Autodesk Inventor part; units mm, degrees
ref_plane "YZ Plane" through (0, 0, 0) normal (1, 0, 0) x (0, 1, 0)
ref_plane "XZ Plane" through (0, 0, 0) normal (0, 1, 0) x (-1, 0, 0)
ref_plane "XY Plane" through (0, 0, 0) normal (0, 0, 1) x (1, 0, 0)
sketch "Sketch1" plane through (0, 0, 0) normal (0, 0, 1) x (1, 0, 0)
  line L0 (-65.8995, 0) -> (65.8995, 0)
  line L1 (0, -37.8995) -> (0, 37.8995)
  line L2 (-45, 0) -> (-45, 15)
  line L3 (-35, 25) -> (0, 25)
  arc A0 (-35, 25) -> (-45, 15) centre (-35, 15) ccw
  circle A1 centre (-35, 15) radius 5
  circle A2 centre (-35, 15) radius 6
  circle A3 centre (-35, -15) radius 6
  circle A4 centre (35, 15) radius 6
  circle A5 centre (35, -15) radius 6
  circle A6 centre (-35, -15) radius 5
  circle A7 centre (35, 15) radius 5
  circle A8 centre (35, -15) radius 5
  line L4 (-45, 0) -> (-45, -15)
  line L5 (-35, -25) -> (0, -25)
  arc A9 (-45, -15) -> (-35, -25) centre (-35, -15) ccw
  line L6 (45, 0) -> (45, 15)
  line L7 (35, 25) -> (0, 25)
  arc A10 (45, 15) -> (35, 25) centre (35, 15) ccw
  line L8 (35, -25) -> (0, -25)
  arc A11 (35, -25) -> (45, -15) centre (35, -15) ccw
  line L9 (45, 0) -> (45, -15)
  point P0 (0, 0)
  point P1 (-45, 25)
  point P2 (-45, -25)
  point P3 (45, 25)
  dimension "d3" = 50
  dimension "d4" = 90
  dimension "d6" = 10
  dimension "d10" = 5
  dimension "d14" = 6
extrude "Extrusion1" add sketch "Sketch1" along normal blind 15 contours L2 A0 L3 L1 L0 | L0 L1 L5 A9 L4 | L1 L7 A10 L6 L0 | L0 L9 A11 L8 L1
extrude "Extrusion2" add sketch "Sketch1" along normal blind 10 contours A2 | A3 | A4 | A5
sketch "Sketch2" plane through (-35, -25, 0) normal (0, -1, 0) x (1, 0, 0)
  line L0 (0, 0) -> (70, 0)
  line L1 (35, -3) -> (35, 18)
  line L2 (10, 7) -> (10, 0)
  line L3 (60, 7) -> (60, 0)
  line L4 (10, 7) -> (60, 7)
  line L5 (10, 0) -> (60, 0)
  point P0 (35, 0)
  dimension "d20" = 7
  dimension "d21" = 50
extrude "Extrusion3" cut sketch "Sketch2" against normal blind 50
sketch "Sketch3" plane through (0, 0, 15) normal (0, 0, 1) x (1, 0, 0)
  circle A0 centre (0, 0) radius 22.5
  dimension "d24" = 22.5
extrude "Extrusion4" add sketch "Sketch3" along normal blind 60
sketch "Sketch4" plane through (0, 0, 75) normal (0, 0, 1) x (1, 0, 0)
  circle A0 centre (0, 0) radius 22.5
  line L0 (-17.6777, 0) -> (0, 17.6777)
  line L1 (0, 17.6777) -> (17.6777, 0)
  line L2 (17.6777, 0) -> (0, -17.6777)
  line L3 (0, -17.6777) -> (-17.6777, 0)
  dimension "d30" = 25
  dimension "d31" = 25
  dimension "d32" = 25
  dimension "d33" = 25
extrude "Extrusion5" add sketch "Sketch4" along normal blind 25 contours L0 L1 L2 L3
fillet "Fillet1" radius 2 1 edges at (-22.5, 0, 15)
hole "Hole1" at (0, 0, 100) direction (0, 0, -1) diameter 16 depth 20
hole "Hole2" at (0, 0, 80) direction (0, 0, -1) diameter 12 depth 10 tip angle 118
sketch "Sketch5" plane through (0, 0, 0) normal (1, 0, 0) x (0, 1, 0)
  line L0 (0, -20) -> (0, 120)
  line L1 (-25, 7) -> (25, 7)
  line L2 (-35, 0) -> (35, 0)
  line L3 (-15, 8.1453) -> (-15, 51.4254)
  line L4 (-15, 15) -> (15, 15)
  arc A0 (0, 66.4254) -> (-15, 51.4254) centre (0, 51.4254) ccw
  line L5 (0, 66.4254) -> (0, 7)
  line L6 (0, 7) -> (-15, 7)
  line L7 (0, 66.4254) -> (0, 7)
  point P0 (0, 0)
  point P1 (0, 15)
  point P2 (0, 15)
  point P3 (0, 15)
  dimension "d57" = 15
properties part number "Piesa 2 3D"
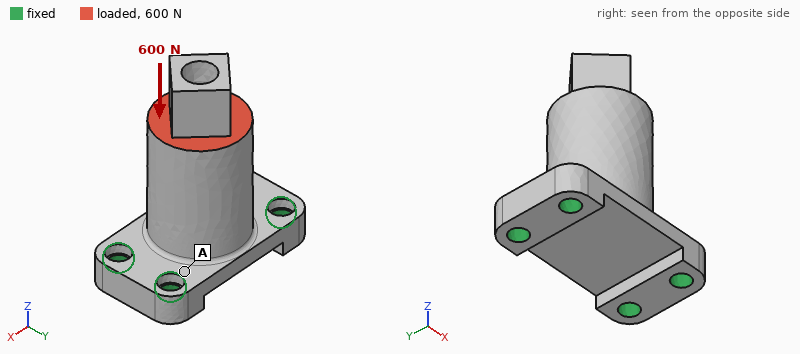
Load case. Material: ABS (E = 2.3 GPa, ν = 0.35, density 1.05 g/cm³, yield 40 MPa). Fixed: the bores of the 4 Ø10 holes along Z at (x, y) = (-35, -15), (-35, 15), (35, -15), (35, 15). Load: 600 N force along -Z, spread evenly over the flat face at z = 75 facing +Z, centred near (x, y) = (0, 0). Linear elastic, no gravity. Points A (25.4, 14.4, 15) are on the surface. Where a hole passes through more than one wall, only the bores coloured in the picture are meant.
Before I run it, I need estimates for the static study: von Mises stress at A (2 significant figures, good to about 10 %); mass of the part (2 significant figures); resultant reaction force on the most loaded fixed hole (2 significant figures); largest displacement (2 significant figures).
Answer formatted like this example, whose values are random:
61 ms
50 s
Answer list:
0.58 MPa
160 g
200 N
39 µm
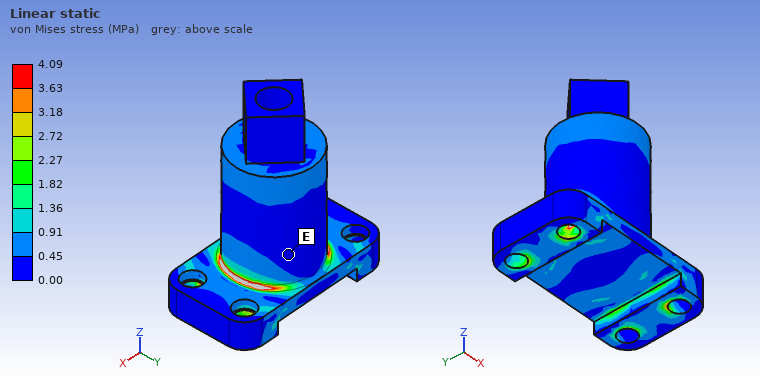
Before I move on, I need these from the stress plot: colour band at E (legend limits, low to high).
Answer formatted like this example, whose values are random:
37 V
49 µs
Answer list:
0.00 to 0.45 MPa
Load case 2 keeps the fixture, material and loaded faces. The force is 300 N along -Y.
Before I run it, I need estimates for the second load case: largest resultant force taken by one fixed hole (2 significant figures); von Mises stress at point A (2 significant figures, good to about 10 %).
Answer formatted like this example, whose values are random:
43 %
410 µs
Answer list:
400 N
4.0 MPa
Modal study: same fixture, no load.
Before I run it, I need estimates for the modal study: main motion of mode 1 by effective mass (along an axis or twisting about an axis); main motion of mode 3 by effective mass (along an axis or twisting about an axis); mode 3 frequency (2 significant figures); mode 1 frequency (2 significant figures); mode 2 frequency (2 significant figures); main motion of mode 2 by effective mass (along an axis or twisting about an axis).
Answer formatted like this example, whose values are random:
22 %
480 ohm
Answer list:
along Y
along Z
1900 Hz
590 Hz
1000 Hz
along X
